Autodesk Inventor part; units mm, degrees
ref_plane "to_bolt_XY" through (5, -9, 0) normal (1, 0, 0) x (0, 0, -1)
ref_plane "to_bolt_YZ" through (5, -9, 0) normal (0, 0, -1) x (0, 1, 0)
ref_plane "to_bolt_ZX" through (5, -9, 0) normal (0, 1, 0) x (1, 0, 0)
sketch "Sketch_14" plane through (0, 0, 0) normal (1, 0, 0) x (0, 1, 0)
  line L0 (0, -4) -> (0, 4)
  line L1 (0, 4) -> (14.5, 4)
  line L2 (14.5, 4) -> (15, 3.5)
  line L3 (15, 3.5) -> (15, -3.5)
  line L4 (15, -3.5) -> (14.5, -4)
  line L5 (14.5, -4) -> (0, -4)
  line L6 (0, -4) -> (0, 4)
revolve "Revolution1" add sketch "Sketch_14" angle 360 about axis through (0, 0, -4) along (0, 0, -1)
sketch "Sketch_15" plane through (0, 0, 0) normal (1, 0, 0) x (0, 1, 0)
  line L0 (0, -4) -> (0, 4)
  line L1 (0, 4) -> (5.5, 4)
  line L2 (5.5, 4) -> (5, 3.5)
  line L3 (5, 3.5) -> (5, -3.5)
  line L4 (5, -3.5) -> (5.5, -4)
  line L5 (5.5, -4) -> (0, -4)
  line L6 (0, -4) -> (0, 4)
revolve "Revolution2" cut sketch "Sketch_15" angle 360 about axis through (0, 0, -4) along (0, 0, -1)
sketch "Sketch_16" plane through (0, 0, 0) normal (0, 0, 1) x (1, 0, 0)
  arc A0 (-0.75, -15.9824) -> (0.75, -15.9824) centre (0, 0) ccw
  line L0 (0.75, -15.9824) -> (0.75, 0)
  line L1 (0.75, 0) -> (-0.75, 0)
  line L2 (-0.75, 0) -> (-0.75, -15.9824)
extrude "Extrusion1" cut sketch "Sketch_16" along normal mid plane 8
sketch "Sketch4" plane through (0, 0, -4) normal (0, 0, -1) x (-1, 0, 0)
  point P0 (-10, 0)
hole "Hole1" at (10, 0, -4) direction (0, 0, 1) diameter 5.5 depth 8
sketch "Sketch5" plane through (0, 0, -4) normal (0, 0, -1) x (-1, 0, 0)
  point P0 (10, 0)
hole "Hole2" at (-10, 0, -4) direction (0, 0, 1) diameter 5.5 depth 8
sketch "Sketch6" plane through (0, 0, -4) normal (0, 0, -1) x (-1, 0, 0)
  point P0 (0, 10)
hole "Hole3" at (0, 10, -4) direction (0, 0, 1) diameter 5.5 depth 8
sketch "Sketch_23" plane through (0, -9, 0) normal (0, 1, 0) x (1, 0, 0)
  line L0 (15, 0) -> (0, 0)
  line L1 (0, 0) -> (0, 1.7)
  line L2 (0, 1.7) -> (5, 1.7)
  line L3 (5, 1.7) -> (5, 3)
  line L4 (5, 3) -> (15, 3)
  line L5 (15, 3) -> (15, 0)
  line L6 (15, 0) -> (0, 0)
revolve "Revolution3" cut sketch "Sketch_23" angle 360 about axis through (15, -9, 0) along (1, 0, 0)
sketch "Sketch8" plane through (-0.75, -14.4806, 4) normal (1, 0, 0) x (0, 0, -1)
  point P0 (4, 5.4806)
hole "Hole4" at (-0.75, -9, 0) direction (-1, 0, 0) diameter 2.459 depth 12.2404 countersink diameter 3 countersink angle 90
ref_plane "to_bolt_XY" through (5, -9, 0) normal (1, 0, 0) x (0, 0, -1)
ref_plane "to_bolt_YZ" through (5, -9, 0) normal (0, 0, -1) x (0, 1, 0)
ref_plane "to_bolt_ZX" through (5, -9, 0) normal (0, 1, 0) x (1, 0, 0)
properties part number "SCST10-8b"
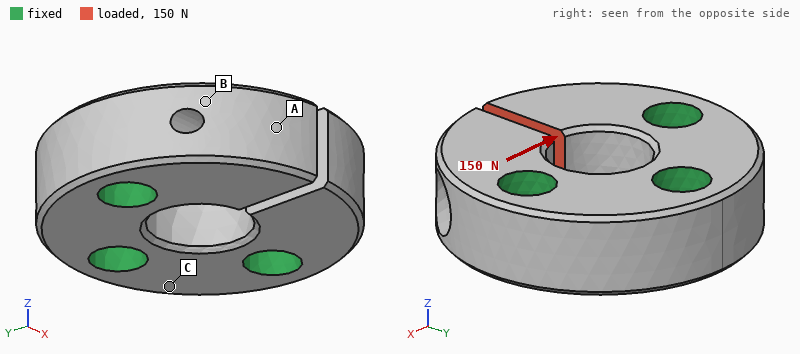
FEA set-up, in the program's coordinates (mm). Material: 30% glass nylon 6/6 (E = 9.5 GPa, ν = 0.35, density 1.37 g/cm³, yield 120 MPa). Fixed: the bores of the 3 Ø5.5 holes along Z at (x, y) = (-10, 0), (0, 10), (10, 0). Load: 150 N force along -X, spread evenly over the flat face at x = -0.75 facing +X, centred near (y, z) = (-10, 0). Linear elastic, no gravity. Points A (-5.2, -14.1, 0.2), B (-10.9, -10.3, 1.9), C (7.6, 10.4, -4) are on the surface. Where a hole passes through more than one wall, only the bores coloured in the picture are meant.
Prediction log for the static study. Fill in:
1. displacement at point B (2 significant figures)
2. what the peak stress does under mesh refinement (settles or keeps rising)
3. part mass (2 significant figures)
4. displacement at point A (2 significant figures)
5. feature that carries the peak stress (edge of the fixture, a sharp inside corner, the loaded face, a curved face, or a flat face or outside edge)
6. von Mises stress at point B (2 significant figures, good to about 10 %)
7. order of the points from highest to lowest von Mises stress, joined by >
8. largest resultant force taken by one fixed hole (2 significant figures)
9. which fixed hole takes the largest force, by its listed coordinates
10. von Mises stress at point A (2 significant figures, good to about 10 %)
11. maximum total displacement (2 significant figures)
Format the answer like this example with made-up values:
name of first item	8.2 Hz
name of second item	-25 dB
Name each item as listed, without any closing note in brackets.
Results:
displacement at point B	13 µm
what the peak stress does under mesh refinement	keeps rising
part mass	5.5 g
displacement at point A	22 µm
feature that carries the peak stress	edge of the fixture
von Mises stress at point B	4.9 MPa
order of the points from highest to lowest von Mises stress, joined by >	B > A > C
largest resultant force taken by one fixed hole	160 N
which fixed hole takes the largest force, by its listed coordinates	(-10, 0)
von Mises stress at point A	2.3 MPa
maximum total displacement	28 µm
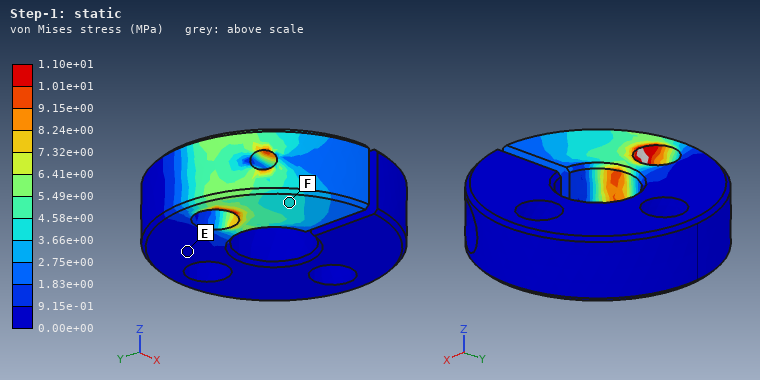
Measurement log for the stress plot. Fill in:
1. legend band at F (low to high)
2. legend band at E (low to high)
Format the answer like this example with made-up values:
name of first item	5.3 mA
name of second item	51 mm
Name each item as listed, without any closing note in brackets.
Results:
legend band at F	3.66e+00 to 4.58e+00 MPa
legend band at E	0.00e+00 to 9.15e-01 MPa
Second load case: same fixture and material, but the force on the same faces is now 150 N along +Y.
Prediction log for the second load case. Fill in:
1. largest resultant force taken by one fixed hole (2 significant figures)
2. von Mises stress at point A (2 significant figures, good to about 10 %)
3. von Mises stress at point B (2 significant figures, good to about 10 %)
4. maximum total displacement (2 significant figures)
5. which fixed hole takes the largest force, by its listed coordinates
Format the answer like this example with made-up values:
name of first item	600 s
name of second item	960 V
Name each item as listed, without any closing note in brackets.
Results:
largest resultant force taken by one fixed hole	130 N
von Mises stress at point A	3.1 MPa
von Mises stress at point B	5.5 MPa
maximum total displacement	33 µm
which fixed hole takes the largest force, by its listed coordinates	(-10, 0)
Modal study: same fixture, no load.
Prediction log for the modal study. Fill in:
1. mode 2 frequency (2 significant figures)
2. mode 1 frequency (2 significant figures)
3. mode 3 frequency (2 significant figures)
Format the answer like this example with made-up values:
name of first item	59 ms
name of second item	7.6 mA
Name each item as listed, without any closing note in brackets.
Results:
mode 2 frequency	15 kHz
mode 1 frequency	13 kHz
mode 3 frequency	16 kHz
